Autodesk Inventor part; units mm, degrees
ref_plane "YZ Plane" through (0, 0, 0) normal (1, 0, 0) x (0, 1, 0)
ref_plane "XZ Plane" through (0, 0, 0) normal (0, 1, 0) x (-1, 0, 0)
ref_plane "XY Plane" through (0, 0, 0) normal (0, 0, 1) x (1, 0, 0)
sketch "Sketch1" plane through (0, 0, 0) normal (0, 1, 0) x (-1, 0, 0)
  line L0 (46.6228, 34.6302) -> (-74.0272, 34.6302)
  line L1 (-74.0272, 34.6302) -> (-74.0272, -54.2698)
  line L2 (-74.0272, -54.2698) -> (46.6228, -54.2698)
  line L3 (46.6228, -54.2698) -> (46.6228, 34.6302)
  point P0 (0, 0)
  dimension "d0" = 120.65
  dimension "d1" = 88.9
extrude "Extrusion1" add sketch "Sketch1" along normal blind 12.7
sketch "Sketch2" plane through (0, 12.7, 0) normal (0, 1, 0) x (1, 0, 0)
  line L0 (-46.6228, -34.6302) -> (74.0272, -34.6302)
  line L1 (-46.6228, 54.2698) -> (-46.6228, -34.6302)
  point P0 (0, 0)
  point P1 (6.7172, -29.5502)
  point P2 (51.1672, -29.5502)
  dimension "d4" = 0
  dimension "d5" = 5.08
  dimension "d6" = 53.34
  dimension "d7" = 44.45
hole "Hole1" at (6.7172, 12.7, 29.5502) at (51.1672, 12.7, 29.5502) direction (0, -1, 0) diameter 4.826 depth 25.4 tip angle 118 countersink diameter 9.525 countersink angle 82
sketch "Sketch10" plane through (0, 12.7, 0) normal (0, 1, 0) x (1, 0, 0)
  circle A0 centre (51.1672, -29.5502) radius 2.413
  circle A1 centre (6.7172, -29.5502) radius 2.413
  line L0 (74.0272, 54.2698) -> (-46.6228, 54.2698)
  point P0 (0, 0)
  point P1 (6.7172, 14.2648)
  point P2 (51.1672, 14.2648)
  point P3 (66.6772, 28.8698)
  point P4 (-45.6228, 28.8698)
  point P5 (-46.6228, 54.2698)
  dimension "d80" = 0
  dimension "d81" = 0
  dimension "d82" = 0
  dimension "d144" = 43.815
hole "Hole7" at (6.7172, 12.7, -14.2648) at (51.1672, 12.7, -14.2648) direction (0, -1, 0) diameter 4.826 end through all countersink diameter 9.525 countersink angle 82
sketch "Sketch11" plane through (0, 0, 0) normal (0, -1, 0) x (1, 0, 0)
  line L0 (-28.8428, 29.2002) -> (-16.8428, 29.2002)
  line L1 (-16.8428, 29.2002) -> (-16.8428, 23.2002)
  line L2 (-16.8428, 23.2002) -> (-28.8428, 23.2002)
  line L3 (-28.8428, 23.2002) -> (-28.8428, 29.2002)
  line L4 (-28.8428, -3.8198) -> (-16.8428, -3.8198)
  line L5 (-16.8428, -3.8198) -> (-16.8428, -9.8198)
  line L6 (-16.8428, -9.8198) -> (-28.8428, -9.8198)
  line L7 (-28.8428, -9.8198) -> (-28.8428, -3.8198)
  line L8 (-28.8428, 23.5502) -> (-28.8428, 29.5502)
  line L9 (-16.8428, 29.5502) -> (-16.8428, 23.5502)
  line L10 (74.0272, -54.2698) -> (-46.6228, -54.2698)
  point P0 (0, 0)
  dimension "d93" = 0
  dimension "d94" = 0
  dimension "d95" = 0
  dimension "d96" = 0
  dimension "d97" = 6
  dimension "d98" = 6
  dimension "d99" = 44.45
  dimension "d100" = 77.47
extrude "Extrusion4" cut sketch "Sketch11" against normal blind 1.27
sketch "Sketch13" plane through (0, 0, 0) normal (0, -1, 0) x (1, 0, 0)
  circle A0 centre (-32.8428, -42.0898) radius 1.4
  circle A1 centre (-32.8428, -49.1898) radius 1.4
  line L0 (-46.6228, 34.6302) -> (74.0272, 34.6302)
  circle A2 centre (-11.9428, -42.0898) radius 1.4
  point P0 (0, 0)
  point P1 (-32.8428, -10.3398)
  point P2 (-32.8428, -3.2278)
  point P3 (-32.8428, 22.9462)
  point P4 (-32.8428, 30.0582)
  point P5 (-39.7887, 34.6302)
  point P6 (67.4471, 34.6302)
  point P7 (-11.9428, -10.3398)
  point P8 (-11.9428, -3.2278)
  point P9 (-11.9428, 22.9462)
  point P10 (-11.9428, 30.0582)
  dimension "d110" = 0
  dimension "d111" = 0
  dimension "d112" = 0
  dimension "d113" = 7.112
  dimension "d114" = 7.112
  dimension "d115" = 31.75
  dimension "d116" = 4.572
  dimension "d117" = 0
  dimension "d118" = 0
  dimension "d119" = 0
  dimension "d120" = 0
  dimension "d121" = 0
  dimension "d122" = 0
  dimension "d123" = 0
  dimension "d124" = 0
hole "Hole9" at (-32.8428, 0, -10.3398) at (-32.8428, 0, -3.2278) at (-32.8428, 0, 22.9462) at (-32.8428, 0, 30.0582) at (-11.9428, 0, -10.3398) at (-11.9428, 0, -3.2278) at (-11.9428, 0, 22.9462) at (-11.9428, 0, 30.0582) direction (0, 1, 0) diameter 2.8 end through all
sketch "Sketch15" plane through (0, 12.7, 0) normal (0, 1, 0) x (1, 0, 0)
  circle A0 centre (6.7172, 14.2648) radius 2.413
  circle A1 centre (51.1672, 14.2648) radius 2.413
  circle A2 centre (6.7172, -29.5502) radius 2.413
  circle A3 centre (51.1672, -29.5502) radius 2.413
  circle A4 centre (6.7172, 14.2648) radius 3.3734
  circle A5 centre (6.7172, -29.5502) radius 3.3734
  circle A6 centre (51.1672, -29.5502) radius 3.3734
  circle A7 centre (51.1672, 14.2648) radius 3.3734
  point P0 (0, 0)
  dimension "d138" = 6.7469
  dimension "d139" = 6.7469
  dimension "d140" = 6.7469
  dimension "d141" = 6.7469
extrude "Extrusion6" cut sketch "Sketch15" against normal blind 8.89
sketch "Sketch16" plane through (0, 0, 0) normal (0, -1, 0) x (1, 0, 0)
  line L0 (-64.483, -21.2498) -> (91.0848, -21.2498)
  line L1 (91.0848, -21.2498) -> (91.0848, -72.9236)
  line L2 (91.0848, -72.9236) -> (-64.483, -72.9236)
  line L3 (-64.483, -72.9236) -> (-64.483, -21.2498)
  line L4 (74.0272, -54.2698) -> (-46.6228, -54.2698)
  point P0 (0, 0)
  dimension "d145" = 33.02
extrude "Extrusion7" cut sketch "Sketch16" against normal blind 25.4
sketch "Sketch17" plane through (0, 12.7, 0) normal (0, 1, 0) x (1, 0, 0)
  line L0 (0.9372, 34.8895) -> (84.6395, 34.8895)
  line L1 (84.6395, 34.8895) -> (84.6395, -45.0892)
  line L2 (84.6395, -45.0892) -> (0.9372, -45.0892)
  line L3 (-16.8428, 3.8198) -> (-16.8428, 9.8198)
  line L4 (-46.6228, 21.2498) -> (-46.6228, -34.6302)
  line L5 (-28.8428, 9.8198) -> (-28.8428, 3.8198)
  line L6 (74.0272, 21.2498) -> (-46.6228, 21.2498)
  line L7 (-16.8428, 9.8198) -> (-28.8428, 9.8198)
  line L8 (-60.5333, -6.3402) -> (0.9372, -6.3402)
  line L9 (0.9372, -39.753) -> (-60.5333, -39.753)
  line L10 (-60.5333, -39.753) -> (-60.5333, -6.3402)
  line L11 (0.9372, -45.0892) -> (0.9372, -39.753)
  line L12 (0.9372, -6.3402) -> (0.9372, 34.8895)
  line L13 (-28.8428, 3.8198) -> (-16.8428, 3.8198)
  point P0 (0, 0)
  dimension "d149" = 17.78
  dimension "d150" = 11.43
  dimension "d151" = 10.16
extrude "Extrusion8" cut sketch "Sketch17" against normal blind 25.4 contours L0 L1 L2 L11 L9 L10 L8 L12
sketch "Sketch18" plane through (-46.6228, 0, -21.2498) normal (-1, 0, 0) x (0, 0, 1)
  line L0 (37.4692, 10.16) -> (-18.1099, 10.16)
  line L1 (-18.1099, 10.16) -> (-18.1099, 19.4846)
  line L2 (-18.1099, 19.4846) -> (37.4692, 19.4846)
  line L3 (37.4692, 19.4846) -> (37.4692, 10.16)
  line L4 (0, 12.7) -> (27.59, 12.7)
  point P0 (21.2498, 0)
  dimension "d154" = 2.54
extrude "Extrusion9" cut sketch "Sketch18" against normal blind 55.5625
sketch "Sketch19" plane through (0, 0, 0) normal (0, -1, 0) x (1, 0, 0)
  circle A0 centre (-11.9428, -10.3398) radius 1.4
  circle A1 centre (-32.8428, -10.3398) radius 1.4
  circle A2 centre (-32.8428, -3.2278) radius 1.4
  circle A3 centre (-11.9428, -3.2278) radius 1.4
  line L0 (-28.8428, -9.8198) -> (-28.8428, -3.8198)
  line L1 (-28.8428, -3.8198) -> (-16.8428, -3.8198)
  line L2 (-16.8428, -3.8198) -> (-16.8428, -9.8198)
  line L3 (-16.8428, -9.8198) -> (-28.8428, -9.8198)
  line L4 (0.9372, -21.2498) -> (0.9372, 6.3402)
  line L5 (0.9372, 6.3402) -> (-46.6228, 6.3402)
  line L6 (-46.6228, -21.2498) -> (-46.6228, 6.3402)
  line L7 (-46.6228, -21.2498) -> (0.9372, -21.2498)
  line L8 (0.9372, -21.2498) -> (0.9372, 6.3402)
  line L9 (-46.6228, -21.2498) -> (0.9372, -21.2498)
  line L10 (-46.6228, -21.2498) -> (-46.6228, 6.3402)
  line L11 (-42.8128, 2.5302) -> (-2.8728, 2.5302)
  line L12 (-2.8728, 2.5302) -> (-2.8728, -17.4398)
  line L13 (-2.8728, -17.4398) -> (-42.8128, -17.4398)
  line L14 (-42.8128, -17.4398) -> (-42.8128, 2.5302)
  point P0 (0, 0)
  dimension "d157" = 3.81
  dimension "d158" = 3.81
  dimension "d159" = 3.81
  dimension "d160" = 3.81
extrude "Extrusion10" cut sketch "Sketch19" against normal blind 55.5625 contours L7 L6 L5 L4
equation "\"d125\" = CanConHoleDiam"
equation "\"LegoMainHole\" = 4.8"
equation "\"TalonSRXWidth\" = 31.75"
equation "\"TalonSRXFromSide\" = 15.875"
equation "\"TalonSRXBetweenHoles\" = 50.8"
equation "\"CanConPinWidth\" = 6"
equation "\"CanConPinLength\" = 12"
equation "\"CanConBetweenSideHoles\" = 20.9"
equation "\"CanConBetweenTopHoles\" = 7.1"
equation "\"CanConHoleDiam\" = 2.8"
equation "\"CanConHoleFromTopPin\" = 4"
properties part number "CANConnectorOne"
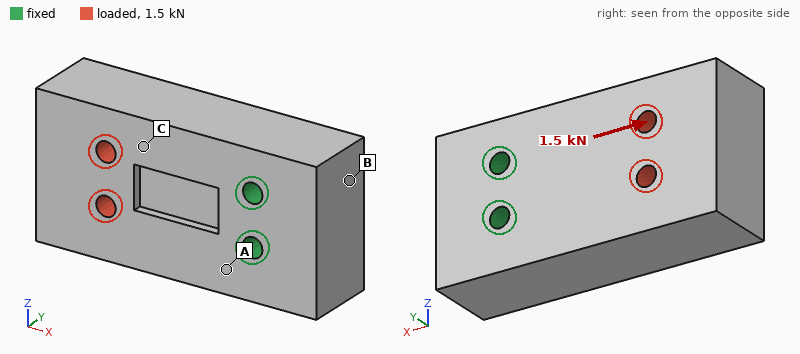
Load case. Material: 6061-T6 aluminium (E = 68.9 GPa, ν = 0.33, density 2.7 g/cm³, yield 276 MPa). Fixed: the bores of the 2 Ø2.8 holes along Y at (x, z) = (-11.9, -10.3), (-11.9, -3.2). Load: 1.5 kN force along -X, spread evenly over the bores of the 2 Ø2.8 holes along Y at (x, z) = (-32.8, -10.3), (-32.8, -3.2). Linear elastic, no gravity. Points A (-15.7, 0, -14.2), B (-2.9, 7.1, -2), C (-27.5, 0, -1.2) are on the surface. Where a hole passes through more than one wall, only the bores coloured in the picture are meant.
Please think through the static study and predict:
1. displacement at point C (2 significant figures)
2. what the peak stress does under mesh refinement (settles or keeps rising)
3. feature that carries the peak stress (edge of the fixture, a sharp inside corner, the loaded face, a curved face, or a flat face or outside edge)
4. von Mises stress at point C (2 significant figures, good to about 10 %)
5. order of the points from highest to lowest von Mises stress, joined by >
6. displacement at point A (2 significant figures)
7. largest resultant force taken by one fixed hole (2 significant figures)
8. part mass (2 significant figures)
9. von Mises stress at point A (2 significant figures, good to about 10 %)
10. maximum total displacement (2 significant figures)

2.3 µm
keeps rising
edge of the fixture
9.2 MPa
C > A > B
0.80 µm
760 N
21 g
5.4 MPa
3.4 µm
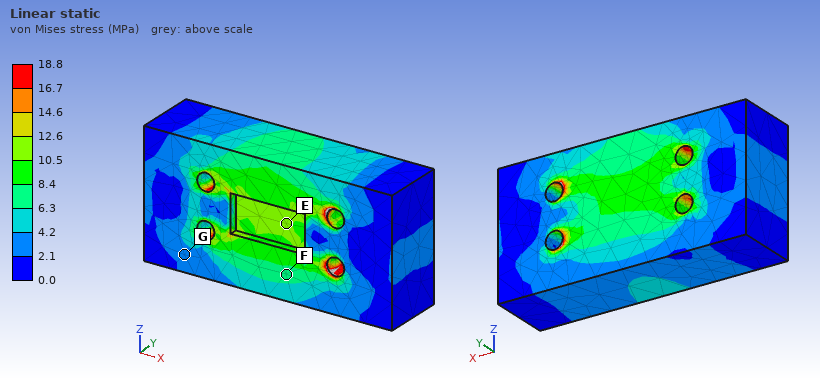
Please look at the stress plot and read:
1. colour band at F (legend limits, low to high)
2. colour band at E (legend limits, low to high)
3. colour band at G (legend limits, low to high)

6.3 to 8.4 MPa
10.5 to 12.6 MPa
2.1 to 4.2 MPa
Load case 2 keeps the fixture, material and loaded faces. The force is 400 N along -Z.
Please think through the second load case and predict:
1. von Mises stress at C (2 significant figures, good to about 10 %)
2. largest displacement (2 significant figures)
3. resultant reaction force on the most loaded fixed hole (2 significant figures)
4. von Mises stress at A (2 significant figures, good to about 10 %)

4.4 MPa
11 µm
910 N
5.5 MPa
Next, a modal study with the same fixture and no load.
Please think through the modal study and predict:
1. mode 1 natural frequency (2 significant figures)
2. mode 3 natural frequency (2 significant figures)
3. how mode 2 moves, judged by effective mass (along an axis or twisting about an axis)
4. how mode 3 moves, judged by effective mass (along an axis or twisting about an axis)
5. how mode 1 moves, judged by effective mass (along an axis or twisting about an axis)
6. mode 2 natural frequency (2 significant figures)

7800 Hz
19 kHz
along Z
twisting about X
along Y
11 kHz
